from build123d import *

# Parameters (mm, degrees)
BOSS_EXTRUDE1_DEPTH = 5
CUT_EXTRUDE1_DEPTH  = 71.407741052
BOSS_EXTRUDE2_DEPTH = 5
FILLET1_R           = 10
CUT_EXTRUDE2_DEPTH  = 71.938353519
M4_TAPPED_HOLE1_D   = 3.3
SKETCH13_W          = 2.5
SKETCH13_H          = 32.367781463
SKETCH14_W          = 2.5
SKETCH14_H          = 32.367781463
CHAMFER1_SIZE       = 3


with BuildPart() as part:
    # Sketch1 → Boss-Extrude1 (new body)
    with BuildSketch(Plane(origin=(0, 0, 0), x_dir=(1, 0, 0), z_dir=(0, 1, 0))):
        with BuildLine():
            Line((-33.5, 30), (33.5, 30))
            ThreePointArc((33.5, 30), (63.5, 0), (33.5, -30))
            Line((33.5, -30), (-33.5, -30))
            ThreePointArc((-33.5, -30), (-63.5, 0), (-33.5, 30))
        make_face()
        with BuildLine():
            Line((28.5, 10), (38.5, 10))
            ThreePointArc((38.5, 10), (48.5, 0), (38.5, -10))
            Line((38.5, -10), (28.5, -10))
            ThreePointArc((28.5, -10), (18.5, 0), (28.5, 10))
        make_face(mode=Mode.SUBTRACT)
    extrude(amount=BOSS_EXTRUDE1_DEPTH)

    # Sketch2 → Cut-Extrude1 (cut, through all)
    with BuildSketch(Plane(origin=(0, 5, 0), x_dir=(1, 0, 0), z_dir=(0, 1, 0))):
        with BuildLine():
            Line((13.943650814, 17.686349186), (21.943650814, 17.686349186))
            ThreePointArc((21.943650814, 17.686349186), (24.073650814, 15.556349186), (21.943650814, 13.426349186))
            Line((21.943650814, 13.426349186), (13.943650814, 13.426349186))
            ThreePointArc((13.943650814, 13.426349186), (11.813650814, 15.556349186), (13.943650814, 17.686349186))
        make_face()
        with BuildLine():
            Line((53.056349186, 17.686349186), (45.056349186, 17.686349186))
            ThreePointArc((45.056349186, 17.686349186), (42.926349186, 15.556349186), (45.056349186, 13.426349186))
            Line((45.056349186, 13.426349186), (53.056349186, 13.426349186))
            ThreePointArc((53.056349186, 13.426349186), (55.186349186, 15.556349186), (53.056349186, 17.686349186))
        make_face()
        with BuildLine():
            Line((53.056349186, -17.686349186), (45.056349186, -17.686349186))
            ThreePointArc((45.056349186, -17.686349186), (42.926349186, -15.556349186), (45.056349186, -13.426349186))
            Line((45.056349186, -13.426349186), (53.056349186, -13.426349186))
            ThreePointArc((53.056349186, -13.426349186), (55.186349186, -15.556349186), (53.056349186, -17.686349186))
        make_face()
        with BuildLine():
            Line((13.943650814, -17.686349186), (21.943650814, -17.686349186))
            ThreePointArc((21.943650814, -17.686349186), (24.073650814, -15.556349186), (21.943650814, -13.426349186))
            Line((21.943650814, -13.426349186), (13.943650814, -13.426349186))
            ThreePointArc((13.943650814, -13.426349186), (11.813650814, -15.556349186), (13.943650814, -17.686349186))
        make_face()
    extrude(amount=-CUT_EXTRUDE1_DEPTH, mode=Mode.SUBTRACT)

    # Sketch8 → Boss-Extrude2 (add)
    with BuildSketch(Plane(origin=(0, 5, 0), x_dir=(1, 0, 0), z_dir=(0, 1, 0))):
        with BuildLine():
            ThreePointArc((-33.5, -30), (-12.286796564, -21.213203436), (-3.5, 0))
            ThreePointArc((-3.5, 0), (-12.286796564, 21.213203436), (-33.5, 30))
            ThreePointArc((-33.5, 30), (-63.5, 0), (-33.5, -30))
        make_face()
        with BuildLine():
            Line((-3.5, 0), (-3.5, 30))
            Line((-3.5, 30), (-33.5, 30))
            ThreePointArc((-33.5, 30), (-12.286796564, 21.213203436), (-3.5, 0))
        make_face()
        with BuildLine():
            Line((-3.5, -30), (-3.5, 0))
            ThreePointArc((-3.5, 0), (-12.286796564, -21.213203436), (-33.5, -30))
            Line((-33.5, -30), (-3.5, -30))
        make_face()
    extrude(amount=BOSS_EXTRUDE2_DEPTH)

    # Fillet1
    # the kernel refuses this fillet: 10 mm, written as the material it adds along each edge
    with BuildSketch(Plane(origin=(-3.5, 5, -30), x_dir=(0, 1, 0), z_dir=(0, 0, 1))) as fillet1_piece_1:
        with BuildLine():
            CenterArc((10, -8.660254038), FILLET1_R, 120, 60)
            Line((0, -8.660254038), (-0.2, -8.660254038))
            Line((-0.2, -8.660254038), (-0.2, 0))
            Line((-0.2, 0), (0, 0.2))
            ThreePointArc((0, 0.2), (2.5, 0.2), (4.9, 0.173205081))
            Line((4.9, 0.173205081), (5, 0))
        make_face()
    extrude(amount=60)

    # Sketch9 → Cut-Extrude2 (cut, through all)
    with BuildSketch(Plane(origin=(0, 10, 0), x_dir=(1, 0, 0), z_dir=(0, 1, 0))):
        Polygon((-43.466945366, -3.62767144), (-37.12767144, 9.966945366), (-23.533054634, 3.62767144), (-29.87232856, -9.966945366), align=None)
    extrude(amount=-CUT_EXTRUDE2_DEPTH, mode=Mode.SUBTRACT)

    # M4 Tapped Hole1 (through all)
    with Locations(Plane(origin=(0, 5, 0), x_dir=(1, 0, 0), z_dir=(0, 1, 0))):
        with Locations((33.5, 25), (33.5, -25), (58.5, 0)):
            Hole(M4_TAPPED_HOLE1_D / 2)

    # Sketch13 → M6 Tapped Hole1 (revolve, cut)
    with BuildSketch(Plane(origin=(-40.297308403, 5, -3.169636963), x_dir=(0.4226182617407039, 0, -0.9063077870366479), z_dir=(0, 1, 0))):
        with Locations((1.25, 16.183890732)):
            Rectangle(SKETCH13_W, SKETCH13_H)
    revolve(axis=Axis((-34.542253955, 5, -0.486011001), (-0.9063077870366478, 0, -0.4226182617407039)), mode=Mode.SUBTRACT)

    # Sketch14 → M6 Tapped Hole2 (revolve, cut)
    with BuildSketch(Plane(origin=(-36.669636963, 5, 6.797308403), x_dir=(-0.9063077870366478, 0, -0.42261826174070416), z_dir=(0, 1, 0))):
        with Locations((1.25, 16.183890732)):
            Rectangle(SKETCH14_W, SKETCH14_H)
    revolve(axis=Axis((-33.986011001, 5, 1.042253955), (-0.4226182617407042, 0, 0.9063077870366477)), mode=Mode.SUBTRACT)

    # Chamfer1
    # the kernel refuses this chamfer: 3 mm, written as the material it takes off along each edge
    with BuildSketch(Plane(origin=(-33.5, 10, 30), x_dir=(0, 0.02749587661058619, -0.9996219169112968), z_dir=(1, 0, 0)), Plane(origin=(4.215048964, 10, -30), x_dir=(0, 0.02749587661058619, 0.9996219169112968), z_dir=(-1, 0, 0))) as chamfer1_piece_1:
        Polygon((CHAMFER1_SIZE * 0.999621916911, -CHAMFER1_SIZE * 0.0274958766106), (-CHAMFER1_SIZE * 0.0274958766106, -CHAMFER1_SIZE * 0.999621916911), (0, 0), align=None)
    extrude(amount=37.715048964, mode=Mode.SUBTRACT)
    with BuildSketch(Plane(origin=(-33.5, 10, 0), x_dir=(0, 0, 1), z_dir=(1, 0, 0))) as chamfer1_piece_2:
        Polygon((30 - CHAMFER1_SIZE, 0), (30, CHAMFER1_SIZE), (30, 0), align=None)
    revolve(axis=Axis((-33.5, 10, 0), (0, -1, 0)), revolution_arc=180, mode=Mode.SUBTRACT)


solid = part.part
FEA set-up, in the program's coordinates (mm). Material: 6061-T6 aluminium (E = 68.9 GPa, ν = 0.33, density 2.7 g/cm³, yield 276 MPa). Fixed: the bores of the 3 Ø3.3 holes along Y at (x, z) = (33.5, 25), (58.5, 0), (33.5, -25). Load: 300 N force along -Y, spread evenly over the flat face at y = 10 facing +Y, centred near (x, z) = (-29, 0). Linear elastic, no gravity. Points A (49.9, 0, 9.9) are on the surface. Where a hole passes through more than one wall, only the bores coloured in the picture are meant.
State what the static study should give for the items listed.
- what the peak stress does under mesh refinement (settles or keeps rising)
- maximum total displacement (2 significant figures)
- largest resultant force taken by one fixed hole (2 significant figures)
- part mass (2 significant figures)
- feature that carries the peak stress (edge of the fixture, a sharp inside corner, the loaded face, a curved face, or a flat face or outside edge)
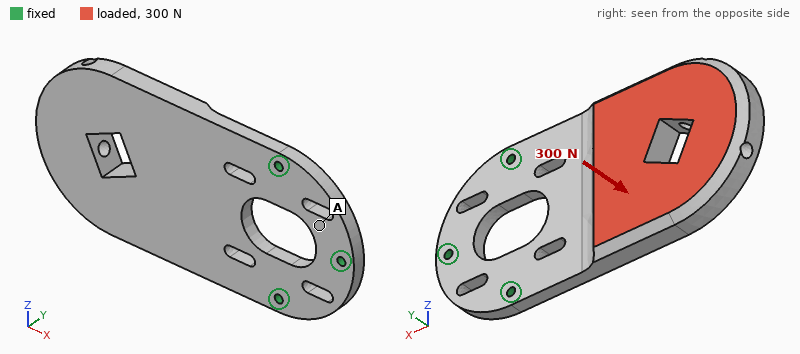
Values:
keeps rising
1.3 mm
250 N
120 g
edge of the fixture
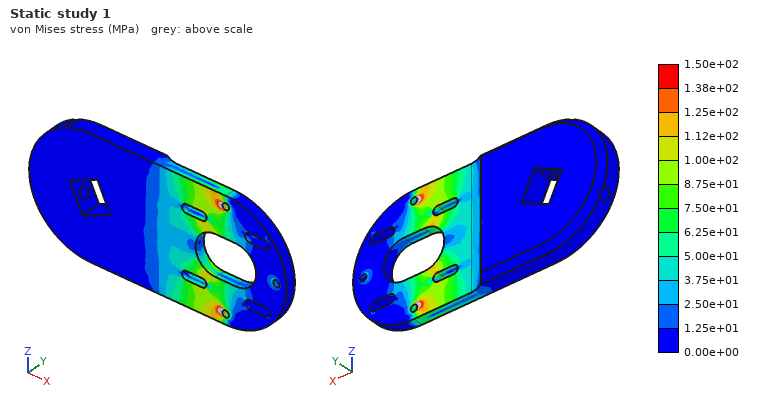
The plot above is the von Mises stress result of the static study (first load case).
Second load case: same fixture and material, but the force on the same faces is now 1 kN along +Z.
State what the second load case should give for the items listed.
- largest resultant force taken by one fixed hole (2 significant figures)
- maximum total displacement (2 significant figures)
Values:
1.3 kN
69 µm
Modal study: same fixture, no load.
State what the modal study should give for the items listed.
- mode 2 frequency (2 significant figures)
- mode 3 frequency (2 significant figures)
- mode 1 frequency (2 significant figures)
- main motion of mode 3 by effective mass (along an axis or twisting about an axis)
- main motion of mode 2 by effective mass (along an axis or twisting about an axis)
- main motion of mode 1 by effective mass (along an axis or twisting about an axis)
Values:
1800 Hz
3300 Hz
330 Hz
along Z
twisting about X
along Y
